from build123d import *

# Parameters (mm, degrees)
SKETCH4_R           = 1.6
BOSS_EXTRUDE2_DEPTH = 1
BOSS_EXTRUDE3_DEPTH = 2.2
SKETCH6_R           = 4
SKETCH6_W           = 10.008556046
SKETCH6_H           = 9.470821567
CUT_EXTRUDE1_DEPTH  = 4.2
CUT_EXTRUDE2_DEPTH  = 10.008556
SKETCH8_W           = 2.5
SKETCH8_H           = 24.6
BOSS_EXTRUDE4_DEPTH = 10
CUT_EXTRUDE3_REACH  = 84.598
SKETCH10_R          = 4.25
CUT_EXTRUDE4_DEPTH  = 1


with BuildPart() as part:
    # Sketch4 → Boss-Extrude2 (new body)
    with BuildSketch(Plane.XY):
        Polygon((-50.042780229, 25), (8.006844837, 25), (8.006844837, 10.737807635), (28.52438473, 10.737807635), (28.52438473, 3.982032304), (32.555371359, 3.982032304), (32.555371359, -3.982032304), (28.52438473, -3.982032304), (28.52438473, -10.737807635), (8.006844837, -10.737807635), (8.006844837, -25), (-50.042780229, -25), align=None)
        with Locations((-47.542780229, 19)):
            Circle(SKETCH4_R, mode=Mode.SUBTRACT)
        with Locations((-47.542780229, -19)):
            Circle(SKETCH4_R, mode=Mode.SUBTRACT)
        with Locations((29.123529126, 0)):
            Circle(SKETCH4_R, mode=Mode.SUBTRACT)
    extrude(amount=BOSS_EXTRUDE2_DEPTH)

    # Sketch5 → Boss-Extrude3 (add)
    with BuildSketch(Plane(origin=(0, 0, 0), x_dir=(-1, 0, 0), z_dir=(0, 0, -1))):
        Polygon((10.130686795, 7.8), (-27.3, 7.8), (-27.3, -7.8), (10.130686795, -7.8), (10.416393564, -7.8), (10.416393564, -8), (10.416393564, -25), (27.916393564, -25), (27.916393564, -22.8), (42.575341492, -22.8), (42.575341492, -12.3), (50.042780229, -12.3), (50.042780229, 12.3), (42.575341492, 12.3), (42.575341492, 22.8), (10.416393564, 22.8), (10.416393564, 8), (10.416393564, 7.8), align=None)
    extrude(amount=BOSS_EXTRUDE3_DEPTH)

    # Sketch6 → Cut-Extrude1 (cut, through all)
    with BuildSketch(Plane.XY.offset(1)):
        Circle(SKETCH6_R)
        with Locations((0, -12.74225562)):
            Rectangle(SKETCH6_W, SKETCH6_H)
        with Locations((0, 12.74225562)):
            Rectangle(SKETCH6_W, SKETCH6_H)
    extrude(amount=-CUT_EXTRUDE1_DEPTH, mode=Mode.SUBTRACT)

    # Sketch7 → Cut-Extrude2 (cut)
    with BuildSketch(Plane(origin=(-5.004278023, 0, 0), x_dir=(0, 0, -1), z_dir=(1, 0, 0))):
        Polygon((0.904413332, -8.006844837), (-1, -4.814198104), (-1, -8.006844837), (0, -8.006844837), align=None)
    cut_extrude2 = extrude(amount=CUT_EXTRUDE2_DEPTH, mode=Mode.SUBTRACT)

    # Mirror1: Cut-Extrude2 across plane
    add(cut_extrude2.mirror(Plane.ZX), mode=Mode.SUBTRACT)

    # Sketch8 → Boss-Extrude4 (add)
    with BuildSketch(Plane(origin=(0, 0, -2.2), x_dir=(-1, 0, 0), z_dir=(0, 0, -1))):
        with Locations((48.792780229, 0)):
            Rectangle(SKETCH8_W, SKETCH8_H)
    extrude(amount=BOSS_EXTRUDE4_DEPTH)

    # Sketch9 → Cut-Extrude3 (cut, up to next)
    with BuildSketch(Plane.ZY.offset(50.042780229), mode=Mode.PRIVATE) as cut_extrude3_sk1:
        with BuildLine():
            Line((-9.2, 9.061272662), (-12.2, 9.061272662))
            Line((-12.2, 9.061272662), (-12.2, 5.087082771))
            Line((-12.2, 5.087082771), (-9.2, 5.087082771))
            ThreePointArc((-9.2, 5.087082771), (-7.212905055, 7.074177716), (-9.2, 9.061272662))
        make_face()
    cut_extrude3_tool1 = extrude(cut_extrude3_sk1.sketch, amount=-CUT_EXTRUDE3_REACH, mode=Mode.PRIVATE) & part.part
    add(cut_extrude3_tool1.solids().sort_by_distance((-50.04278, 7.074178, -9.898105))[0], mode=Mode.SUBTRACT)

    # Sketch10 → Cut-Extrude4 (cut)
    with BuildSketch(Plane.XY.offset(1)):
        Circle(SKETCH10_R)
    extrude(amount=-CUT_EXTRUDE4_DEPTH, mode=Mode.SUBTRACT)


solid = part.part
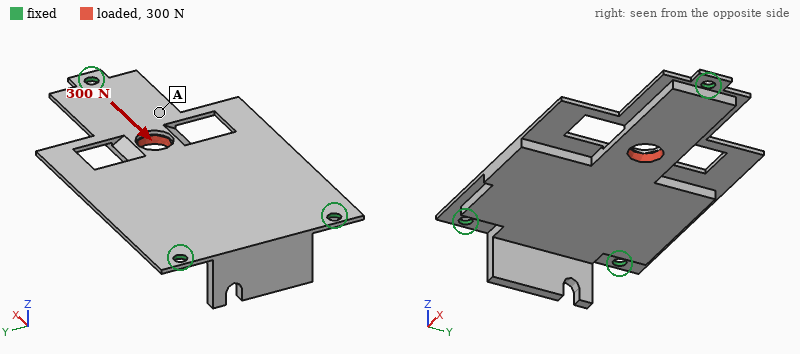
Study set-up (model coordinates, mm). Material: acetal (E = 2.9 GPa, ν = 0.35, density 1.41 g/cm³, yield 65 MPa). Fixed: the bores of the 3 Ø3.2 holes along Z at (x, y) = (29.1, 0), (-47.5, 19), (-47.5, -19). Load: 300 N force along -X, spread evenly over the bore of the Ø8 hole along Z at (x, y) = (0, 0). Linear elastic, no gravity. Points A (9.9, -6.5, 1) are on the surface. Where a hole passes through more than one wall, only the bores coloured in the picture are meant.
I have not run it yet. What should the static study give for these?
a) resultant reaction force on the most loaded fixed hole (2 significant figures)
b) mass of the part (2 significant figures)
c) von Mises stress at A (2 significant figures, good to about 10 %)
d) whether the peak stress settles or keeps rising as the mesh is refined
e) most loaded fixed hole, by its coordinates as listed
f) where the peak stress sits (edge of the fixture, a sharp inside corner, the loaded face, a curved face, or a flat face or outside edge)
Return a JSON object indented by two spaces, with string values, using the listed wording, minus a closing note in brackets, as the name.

{
  "resultant reaction force on the most loaded fixed hole": "140 N",
  "mass of the part": "12 g",
  "von Mises stress at A": "2.5 MPa",
  "whether the peak stress settles or keeps rising as the mesh is refined": "keeps rising",
  "most loaded fixed hole, by its coordinates as listed": "(29.1, 0)",
  "where the peak stress sits": "edge of the fixture"
}
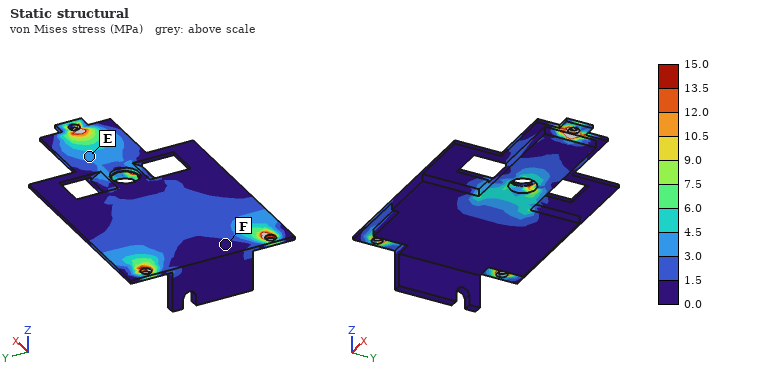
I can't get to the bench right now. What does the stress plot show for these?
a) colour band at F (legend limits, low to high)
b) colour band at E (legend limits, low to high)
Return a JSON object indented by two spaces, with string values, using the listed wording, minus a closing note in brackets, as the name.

{
  "colour band at F": "0.0 to 1.5 MPa",
  "colour band at E": "3.0 to 4.5 MPa"
}
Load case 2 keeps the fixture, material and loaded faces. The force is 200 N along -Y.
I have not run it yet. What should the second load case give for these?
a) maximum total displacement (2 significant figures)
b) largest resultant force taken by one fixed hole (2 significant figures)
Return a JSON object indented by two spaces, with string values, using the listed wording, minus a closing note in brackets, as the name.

{
  "maximum total displacement": "0.23 mm",
  "largest resultant force taken by one fixed hole": "140 N"
}
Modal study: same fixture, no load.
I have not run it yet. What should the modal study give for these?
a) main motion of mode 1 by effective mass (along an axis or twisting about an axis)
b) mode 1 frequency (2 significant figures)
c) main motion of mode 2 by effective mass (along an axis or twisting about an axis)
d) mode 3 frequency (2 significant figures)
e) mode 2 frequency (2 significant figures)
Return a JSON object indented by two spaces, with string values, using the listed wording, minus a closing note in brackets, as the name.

{
  "main motion of mode 1 by effective mass": "along Z",
  "mode 1 frequency": "390 Hz",
  "main motion of mode 2 by effective mass": "twisting about X",
  "mode 3 frequency": "1200 Hz",
  "mode 2 frequency": "720 Hz"
}
